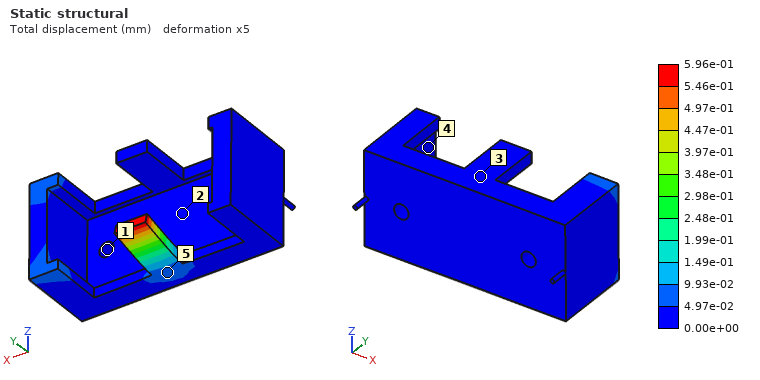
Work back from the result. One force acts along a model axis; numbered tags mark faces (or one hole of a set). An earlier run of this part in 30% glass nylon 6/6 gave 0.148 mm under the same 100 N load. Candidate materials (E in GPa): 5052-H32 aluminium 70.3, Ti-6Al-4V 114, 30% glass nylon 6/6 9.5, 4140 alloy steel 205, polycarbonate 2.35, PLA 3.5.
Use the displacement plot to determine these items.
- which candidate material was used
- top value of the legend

polycarbonate
5.96e-01 mm
